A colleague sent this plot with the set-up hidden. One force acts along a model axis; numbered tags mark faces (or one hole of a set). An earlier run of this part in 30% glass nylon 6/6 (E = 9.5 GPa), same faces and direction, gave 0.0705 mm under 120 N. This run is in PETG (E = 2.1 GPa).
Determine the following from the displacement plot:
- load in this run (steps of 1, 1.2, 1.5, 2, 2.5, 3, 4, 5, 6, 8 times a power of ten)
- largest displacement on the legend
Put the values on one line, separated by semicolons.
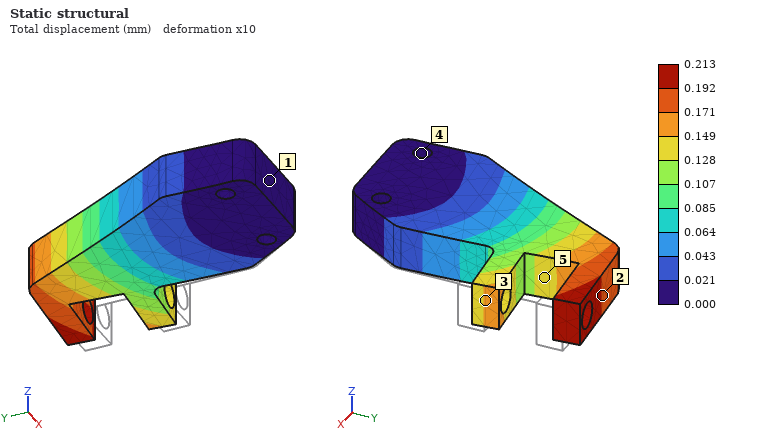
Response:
80 N; 0.213 mm
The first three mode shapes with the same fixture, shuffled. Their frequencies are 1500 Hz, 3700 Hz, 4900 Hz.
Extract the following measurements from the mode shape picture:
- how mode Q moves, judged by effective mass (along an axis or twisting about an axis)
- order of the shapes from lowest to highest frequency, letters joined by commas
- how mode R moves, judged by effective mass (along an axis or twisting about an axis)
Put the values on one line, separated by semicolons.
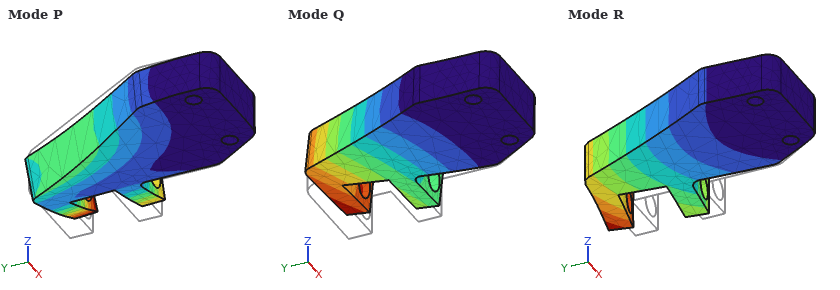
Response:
along Z; Q, R, P; along X
